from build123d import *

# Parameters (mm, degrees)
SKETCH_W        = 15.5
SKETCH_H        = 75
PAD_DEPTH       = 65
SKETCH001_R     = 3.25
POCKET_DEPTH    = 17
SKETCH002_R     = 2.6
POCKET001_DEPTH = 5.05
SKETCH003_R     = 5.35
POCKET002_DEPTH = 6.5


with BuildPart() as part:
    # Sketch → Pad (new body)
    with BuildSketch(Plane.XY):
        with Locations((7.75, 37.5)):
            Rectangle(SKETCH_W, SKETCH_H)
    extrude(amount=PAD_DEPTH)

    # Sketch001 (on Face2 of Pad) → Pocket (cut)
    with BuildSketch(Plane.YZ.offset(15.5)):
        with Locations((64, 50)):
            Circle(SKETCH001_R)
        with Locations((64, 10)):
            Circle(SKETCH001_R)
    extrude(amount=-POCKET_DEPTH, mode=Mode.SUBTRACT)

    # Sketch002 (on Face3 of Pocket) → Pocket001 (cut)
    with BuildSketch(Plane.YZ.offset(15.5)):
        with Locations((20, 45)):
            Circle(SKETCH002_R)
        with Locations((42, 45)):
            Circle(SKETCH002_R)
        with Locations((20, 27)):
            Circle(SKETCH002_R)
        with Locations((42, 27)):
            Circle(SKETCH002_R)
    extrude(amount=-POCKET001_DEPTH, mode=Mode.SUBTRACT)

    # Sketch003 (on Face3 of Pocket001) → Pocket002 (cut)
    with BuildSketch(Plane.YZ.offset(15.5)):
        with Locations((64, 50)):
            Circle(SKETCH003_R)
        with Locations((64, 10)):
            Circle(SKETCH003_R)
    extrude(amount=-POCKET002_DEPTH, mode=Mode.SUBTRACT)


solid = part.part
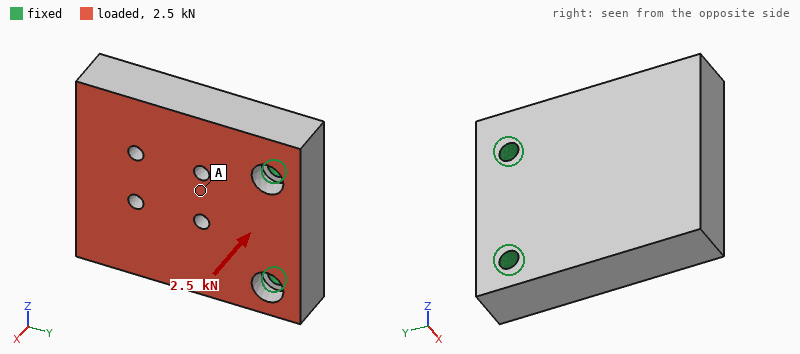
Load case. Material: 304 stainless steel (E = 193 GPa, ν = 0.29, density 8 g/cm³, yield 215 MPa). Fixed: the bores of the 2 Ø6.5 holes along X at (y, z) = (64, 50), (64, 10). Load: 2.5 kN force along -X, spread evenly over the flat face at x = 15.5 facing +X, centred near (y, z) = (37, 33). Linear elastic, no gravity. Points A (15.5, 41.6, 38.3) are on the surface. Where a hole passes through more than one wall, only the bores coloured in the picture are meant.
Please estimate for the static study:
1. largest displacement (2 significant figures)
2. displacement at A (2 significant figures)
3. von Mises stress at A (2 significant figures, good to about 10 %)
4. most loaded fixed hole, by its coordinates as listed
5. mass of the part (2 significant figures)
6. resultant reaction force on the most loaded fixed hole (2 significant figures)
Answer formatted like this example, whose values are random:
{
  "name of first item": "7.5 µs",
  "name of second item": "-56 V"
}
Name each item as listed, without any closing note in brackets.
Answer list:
{
  "largest displacement": "43 µm",
  "displacement at A": "14 µm",
  "von Mises stress at A": "12 MPa",
  "most loaded fixed hole, by its coordinates as listed": "(64, 50)",
  "mass of the part": "590 g",
  "resultant reaction force on the most loaded fixed hole": "1.4 kN"
}
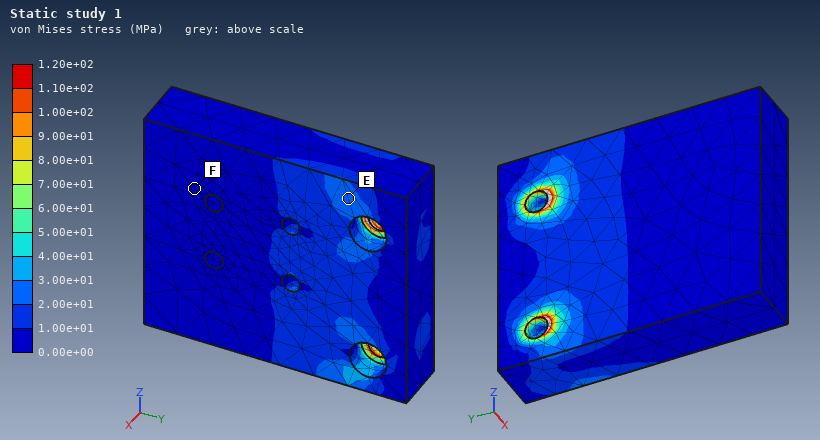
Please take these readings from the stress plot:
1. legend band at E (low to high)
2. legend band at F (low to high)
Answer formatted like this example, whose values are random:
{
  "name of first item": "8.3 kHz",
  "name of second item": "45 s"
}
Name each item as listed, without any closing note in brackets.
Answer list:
{
  "legend band at E": "2.00e+01 to 3.00e+01 MPa",
  "legend band at F": "0.00e+00 to 1.00e+01 MPa"
}
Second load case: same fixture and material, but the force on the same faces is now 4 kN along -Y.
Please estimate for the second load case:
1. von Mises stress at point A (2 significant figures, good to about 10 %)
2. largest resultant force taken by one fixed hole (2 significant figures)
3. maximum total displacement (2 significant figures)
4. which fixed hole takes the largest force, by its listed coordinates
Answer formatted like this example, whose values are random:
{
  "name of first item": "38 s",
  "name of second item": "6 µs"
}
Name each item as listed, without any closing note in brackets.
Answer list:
{
  "von Mises stress at point A": "9.1 MPa",
  "largest resultant force taken by one fixed hole": "2.2 kN",
  "maximum total displacement": "26 µm",
  "which fixed hole takes the largest force, by its listed coordinates": "(64, 50)"
}
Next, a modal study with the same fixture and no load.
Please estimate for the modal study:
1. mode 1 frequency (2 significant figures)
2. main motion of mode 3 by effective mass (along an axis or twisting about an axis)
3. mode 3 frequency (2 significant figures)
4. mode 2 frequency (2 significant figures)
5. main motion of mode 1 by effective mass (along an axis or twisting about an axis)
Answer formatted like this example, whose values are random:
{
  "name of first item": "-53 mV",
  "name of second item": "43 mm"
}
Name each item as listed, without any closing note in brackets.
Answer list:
{
  "mode 1 frequency": "2000 Hz",
  "main motion of mode 3 by effective mass": "along Z",
  "mode 3 frequency": "6600 Hz",
  "mode 2 frequency": "5400 Hz",
  "main motion of mode 1 by effective mass": "along X"
}
